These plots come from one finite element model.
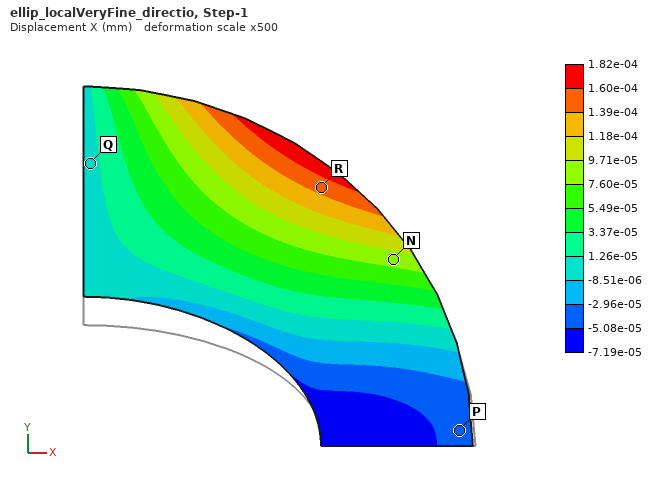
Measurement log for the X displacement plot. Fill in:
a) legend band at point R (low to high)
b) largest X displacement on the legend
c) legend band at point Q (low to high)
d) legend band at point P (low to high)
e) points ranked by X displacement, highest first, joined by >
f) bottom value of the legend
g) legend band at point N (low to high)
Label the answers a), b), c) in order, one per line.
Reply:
a) 1.39e-04 to 1.60e-04 mm
b) 1.82e-04 mm
c) -8.51e-06 to 1.26e-05 mm
d) -5.08e-05 to -2.96e-05 mm
e) R > N > Q > P
f) -7.19e-05 mm
g) 7.60e-05 to 9.71e-05 mm
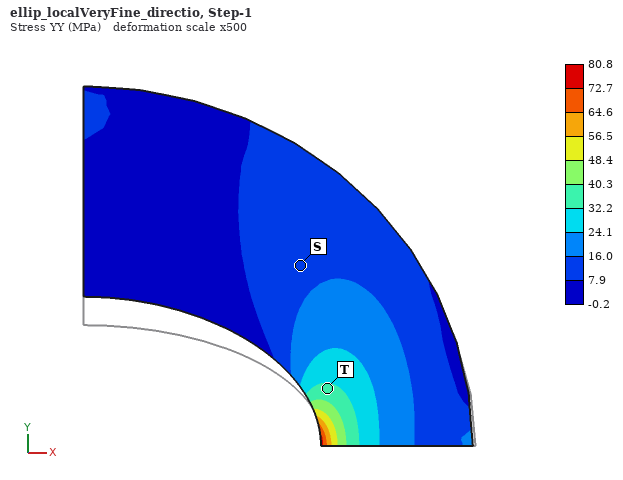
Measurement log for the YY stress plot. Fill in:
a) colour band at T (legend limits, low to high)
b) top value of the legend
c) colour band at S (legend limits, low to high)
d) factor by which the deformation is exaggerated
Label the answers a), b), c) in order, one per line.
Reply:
a) 32.2 to 40.3 MPa
b) 80.8 MPa
c) 7.9 to 16.0 MPa
d) 500
